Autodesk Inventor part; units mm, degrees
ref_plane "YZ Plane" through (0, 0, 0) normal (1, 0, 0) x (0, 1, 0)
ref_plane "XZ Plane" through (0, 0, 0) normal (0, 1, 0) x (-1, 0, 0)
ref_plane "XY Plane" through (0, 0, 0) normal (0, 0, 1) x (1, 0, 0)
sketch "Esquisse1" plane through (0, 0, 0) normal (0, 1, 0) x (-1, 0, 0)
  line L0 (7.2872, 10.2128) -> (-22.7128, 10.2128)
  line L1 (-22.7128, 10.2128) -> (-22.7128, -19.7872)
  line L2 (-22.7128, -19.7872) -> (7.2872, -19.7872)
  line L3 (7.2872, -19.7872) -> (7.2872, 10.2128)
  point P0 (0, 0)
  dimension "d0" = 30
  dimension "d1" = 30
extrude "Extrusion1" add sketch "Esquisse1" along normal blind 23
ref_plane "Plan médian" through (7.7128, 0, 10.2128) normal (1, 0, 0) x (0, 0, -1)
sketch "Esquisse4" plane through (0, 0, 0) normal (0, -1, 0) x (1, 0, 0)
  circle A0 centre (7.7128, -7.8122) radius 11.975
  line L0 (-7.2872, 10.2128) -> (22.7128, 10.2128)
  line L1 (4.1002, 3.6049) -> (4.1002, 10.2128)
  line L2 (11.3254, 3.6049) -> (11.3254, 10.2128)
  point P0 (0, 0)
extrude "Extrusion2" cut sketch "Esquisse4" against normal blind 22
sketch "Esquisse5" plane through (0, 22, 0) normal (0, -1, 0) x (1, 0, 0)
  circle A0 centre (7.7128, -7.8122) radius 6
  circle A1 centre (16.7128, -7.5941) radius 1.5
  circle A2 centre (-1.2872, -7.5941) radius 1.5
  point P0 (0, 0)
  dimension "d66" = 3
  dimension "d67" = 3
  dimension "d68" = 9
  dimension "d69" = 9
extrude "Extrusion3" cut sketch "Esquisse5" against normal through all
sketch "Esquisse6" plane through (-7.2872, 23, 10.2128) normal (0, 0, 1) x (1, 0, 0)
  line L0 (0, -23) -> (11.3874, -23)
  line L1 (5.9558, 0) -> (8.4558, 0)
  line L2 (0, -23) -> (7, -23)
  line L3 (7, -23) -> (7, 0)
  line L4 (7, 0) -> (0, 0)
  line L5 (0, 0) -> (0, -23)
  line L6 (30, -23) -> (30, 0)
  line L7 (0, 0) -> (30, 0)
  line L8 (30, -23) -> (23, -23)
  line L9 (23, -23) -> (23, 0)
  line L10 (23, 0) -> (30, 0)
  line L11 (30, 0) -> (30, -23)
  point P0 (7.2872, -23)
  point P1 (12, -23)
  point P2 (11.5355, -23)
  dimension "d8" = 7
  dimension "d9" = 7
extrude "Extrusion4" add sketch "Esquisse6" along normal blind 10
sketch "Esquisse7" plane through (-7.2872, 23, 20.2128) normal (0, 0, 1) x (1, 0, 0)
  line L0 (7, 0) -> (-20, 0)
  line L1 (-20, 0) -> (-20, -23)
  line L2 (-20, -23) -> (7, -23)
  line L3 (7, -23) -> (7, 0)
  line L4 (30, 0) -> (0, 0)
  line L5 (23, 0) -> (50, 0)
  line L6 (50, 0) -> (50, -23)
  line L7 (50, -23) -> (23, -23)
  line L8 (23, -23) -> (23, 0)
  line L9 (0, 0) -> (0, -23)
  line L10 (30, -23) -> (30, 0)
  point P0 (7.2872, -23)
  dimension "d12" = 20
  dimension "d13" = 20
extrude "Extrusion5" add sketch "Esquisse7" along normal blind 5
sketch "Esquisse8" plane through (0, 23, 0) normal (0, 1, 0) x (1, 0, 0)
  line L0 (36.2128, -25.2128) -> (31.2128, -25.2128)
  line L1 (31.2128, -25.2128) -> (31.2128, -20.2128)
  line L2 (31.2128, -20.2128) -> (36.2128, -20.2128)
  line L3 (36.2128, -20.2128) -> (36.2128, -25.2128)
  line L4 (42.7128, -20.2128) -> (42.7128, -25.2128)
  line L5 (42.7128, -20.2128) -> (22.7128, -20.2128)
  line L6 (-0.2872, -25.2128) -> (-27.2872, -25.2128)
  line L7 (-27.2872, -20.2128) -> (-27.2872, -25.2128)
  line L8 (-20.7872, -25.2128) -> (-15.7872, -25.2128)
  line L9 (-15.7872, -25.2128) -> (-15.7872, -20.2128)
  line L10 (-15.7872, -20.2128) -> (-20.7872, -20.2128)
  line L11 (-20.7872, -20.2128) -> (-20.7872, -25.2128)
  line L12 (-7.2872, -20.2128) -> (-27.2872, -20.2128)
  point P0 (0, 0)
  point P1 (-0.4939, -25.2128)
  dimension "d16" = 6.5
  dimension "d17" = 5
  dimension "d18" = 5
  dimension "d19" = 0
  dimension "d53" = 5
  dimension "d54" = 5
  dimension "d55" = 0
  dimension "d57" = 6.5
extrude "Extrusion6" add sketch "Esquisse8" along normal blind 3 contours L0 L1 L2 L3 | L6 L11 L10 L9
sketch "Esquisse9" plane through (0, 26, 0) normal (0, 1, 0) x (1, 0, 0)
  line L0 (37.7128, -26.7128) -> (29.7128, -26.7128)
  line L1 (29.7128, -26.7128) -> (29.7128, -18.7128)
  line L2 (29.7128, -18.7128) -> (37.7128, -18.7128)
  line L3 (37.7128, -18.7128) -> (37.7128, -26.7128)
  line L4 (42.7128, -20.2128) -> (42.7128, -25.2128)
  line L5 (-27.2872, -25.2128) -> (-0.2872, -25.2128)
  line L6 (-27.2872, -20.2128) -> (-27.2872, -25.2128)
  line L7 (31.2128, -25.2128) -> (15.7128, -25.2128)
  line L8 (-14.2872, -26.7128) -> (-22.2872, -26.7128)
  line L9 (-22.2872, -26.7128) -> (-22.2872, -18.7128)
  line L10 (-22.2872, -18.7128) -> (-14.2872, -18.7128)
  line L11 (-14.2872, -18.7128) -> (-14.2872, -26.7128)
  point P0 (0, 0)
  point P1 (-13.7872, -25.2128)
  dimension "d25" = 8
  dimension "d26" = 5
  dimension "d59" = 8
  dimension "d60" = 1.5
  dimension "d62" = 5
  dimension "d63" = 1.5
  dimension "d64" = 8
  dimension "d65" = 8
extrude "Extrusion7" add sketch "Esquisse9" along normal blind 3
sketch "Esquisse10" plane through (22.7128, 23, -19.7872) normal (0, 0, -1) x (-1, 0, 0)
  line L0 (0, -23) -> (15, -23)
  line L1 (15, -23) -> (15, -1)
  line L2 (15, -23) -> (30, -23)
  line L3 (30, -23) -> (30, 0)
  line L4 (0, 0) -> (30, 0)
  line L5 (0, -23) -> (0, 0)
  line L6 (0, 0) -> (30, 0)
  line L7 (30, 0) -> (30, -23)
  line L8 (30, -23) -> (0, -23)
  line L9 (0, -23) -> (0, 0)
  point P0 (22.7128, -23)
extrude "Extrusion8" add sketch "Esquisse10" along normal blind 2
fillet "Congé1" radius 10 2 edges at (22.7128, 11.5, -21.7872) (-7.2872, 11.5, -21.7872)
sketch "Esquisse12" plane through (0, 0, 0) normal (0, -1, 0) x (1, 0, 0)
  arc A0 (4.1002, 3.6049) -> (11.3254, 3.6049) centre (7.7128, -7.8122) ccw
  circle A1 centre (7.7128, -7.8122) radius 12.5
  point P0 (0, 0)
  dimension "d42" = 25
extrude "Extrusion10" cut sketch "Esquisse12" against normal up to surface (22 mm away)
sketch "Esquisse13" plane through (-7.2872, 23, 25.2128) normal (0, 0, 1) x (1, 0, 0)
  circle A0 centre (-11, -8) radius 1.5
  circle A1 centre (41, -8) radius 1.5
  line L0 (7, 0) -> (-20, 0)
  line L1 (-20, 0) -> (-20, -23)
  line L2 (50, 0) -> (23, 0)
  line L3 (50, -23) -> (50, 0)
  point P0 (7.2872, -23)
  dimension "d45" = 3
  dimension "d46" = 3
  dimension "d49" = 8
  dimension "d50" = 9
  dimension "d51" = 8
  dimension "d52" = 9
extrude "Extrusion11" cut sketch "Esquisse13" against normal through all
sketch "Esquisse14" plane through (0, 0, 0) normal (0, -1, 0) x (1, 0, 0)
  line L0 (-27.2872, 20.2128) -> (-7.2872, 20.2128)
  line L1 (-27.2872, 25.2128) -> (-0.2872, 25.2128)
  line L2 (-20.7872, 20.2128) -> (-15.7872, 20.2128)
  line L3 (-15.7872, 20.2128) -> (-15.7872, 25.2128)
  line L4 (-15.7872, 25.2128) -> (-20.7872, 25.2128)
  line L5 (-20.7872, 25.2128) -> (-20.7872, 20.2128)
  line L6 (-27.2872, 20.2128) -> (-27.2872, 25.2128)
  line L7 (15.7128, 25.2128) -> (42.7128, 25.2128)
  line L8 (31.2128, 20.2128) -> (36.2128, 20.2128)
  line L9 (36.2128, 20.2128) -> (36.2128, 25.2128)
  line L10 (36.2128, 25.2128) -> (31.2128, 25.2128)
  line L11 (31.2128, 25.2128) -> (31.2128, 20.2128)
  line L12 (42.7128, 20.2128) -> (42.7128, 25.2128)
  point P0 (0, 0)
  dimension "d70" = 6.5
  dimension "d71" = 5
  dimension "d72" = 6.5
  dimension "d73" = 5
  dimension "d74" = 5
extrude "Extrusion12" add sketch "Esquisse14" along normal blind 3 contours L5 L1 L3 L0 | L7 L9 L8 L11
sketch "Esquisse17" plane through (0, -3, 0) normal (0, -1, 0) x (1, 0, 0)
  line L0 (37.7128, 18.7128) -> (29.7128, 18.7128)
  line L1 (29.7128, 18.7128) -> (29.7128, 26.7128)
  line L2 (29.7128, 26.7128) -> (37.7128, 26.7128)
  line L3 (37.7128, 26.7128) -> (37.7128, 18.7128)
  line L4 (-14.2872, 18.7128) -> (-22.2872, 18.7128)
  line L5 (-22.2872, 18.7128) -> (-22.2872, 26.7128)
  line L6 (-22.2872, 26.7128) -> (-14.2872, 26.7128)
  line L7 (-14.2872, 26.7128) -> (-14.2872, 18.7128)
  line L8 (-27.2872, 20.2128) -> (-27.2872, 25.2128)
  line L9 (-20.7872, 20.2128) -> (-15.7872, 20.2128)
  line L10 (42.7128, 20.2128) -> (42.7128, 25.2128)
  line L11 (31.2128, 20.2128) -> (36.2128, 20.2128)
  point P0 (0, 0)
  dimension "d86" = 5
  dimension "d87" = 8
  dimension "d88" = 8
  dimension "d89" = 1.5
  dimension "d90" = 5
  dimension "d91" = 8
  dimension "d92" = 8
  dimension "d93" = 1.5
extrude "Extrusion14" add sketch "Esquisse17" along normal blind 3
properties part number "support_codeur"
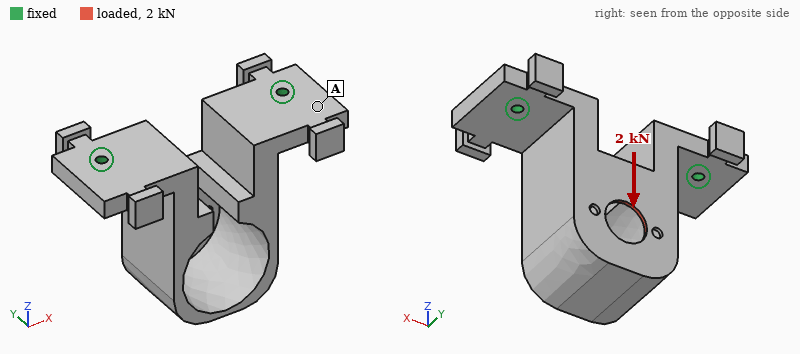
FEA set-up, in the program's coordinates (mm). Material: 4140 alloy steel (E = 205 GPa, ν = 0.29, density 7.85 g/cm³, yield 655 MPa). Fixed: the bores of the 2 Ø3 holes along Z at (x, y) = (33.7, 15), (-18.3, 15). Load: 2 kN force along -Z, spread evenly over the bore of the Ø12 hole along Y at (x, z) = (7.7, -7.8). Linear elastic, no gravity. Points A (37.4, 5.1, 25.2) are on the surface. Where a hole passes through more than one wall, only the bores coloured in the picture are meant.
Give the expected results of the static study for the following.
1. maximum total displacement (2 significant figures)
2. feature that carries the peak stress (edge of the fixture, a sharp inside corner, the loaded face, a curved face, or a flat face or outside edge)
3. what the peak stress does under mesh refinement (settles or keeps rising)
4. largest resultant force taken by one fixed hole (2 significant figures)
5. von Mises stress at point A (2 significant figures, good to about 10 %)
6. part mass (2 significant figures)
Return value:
87 µm
edge of the fixture
keeps rising
1.1 kN
22 MPa
150 g
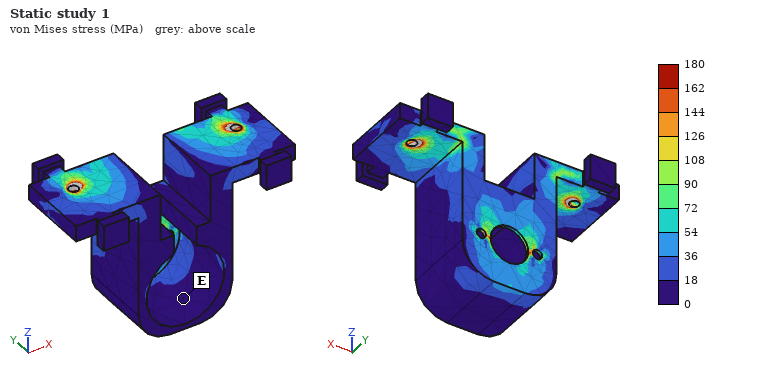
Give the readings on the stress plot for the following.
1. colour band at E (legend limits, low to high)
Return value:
0 to 18 MPa
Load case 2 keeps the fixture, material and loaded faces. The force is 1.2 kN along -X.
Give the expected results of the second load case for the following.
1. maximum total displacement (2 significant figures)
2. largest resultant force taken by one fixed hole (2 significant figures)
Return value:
34 µm
1.0 kN
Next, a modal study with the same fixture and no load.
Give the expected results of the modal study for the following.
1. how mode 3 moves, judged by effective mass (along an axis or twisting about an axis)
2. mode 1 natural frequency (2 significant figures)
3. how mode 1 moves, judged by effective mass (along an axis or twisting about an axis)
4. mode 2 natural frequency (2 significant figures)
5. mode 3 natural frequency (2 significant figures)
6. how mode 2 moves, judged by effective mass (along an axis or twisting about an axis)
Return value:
along Z
1900 Hz
along Y
3500 Hz
5000 Hz
along X
